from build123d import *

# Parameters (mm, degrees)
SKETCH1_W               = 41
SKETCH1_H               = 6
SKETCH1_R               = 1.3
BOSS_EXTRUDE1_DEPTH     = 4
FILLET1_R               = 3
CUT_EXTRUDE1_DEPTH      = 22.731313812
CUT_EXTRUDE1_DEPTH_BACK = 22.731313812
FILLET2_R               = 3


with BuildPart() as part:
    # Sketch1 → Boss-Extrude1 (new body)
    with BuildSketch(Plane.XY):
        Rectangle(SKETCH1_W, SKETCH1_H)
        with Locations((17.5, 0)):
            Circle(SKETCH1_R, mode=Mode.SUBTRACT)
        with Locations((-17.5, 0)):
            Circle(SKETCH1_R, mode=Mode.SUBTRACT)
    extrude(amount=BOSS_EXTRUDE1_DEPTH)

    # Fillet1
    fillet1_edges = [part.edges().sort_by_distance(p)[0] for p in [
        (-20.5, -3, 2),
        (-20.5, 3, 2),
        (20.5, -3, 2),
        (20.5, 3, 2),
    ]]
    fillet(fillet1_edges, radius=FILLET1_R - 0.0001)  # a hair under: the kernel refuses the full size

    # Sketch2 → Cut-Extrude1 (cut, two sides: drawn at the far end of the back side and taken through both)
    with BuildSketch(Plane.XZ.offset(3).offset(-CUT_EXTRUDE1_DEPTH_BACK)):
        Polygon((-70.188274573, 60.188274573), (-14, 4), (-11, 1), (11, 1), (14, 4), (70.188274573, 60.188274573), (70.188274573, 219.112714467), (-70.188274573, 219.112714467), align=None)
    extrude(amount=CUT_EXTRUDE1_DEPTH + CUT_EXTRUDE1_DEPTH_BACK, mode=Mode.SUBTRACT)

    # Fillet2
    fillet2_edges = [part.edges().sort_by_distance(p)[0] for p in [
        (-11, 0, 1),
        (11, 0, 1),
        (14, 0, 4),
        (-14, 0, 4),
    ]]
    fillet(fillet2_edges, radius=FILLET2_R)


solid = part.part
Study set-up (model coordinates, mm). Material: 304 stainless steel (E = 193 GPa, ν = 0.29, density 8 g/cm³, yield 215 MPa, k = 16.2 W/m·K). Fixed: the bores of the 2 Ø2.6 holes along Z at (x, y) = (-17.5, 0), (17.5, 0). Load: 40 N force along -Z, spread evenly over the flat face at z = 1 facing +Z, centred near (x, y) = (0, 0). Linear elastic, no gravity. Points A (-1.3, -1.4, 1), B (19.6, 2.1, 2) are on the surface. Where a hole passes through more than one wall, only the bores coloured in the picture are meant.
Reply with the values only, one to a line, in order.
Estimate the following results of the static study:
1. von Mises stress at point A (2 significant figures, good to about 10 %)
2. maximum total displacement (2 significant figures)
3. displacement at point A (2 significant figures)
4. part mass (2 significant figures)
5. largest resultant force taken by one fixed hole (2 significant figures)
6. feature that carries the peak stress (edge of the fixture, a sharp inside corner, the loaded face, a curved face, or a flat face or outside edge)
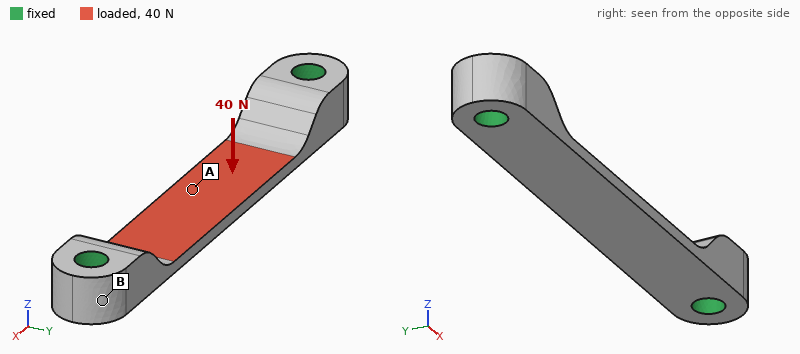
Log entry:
37 MPa
16 µm
15 µm
3.7 g
32 N
a curved face
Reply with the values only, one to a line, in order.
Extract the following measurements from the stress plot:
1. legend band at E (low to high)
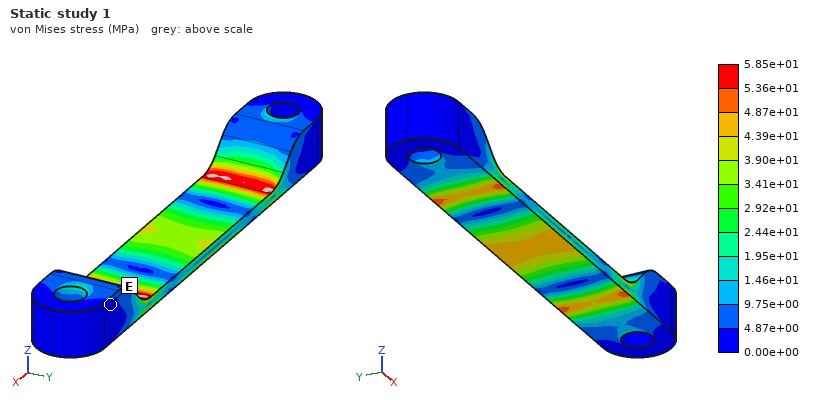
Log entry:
0.00e+00 to 4.87e+00 MPa
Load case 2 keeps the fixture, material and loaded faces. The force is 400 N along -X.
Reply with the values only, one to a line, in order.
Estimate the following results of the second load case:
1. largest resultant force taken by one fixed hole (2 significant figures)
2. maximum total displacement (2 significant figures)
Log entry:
200 N
2.9 µm
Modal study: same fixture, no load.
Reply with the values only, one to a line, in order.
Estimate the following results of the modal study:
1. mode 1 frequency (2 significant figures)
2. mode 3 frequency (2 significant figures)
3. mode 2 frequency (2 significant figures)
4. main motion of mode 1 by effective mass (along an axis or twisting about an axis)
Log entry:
9500 Hz
24 kHz
23 kHz
along Z
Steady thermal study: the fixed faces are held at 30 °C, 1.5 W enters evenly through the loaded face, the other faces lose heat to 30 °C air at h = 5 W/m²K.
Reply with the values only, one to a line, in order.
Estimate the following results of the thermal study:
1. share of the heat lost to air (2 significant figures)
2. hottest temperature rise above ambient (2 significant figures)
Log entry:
3.3 %
63 K
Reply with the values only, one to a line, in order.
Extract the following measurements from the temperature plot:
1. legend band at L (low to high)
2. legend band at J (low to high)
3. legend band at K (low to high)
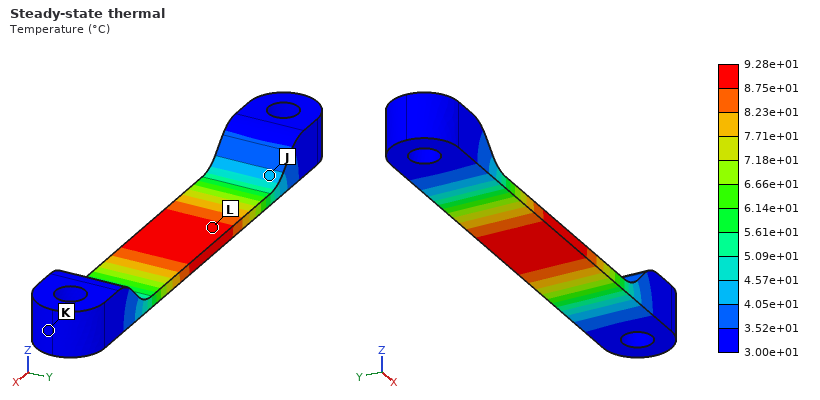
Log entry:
8.75e+01 to 9.28e+01 °C
4.05e+01 to 4.57e+01 °C
3.00e+01 to 3.52e+01 °C
